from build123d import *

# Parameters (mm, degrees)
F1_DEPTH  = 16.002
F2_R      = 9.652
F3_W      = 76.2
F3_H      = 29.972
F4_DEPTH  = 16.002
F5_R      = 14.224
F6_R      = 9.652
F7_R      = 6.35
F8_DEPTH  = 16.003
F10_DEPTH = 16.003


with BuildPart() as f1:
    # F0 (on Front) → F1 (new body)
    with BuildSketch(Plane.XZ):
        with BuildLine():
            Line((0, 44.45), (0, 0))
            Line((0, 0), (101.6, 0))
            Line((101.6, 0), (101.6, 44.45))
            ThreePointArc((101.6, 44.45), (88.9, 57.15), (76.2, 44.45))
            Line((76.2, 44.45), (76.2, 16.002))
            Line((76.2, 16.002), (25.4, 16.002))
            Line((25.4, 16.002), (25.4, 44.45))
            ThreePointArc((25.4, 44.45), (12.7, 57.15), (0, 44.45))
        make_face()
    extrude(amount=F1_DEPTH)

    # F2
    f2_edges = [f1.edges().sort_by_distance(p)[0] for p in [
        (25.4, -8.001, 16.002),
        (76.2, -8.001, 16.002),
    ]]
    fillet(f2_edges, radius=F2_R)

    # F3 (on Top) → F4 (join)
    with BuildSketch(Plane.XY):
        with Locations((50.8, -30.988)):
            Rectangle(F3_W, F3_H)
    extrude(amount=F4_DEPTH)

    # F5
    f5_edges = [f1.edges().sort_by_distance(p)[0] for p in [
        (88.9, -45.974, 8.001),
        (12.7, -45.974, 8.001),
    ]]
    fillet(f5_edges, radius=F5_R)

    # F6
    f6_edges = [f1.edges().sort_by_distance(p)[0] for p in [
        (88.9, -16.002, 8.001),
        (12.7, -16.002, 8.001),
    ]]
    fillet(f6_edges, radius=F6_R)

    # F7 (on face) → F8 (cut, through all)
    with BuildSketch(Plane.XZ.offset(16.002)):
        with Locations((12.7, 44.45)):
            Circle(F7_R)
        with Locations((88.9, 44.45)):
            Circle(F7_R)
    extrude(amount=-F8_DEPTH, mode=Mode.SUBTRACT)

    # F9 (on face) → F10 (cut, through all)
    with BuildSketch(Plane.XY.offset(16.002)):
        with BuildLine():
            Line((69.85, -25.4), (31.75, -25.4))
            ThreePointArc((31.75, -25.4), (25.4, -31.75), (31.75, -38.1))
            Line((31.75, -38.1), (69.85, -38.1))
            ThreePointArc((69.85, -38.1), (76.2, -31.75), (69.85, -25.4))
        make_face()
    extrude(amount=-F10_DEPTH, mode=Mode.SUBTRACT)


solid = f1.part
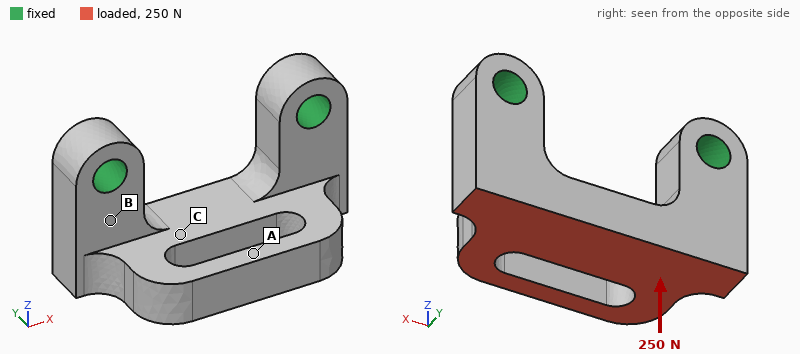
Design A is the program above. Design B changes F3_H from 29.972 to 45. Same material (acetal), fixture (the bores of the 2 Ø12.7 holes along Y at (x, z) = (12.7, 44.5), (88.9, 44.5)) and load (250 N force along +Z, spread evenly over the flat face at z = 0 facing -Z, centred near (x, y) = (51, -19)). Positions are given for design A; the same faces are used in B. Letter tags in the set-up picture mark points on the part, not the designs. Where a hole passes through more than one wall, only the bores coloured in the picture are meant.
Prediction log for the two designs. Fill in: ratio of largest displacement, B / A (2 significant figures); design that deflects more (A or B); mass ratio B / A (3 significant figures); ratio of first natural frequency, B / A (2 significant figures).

1.6
B
1.11
0.80
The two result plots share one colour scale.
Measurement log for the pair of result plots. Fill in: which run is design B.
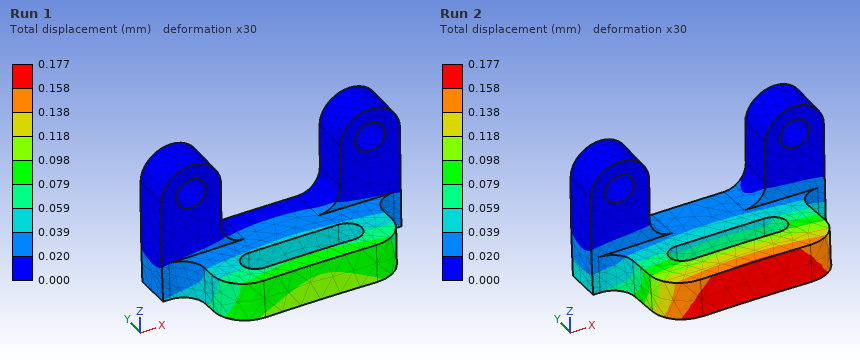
Run 2
